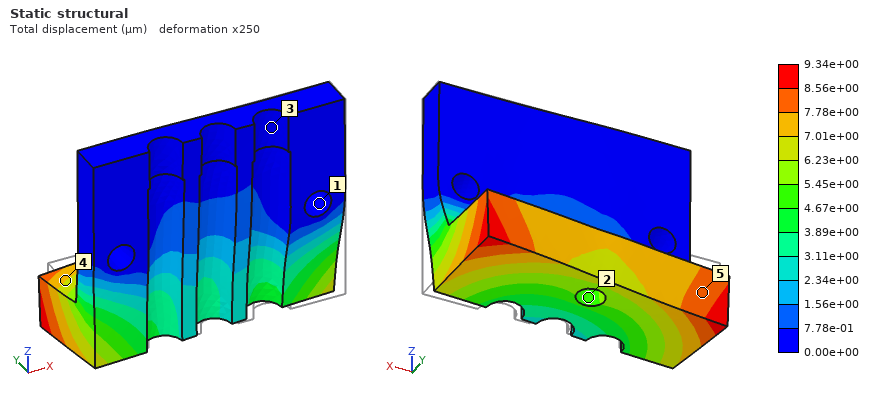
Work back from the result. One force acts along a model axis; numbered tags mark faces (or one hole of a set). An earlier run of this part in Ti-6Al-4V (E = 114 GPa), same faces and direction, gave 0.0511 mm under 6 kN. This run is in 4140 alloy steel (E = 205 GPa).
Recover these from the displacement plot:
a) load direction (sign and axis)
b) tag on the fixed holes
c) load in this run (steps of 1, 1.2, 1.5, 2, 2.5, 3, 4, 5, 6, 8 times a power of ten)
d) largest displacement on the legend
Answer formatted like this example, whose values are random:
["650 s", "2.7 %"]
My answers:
["-X", "1", "2 kN", "9.34e+00 µm"]
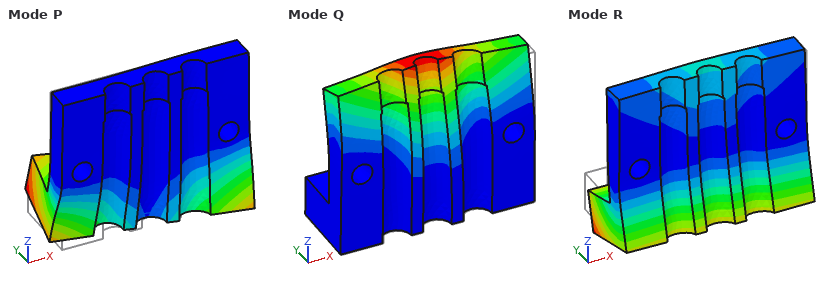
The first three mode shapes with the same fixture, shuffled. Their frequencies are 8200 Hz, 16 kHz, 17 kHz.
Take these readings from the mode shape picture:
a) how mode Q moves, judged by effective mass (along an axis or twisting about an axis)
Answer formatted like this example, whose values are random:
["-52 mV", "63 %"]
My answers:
["along Y"]
